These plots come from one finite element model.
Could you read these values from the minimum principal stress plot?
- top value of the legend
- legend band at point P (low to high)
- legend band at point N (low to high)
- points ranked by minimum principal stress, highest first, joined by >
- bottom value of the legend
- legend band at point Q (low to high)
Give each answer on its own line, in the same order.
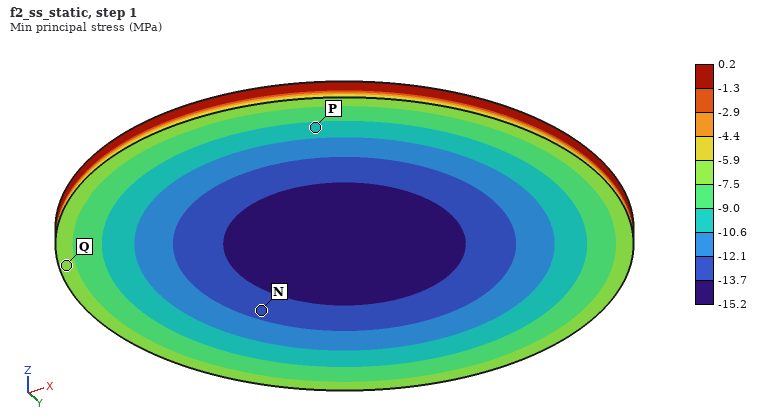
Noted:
0.2 MPa
-10.6 to -9.0 MPa
-13.7 to -12.1 MPa
Q > P > N
-15.2 MPa
-7.5 to -5.9 MPa
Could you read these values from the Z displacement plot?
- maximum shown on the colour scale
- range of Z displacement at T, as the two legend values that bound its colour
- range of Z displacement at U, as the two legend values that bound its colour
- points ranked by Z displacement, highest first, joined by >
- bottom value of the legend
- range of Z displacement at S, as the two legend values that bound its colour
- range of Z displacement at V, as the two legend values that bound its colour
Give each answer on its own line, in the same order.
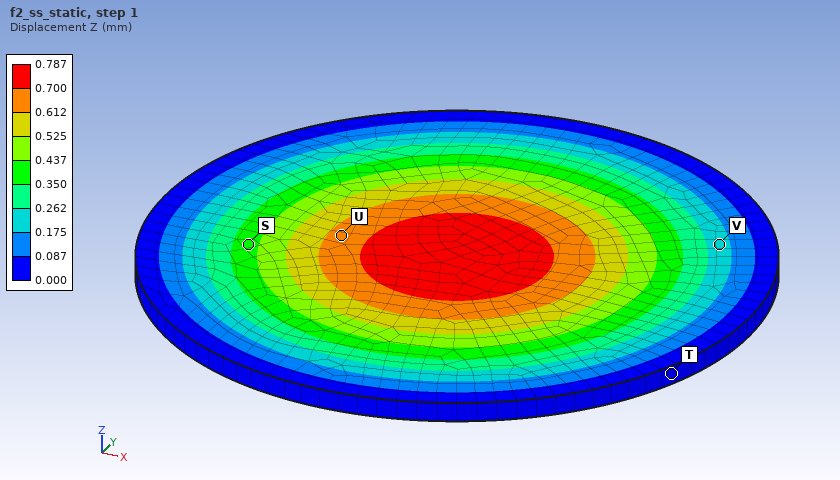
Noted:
0.787 mm
0.000 to 0.087 mm
0.612 to 0.700 mm
U > S > V > T
0.000 mm
0.350 to 0.437 mm
0.175 to 0.262 mm
